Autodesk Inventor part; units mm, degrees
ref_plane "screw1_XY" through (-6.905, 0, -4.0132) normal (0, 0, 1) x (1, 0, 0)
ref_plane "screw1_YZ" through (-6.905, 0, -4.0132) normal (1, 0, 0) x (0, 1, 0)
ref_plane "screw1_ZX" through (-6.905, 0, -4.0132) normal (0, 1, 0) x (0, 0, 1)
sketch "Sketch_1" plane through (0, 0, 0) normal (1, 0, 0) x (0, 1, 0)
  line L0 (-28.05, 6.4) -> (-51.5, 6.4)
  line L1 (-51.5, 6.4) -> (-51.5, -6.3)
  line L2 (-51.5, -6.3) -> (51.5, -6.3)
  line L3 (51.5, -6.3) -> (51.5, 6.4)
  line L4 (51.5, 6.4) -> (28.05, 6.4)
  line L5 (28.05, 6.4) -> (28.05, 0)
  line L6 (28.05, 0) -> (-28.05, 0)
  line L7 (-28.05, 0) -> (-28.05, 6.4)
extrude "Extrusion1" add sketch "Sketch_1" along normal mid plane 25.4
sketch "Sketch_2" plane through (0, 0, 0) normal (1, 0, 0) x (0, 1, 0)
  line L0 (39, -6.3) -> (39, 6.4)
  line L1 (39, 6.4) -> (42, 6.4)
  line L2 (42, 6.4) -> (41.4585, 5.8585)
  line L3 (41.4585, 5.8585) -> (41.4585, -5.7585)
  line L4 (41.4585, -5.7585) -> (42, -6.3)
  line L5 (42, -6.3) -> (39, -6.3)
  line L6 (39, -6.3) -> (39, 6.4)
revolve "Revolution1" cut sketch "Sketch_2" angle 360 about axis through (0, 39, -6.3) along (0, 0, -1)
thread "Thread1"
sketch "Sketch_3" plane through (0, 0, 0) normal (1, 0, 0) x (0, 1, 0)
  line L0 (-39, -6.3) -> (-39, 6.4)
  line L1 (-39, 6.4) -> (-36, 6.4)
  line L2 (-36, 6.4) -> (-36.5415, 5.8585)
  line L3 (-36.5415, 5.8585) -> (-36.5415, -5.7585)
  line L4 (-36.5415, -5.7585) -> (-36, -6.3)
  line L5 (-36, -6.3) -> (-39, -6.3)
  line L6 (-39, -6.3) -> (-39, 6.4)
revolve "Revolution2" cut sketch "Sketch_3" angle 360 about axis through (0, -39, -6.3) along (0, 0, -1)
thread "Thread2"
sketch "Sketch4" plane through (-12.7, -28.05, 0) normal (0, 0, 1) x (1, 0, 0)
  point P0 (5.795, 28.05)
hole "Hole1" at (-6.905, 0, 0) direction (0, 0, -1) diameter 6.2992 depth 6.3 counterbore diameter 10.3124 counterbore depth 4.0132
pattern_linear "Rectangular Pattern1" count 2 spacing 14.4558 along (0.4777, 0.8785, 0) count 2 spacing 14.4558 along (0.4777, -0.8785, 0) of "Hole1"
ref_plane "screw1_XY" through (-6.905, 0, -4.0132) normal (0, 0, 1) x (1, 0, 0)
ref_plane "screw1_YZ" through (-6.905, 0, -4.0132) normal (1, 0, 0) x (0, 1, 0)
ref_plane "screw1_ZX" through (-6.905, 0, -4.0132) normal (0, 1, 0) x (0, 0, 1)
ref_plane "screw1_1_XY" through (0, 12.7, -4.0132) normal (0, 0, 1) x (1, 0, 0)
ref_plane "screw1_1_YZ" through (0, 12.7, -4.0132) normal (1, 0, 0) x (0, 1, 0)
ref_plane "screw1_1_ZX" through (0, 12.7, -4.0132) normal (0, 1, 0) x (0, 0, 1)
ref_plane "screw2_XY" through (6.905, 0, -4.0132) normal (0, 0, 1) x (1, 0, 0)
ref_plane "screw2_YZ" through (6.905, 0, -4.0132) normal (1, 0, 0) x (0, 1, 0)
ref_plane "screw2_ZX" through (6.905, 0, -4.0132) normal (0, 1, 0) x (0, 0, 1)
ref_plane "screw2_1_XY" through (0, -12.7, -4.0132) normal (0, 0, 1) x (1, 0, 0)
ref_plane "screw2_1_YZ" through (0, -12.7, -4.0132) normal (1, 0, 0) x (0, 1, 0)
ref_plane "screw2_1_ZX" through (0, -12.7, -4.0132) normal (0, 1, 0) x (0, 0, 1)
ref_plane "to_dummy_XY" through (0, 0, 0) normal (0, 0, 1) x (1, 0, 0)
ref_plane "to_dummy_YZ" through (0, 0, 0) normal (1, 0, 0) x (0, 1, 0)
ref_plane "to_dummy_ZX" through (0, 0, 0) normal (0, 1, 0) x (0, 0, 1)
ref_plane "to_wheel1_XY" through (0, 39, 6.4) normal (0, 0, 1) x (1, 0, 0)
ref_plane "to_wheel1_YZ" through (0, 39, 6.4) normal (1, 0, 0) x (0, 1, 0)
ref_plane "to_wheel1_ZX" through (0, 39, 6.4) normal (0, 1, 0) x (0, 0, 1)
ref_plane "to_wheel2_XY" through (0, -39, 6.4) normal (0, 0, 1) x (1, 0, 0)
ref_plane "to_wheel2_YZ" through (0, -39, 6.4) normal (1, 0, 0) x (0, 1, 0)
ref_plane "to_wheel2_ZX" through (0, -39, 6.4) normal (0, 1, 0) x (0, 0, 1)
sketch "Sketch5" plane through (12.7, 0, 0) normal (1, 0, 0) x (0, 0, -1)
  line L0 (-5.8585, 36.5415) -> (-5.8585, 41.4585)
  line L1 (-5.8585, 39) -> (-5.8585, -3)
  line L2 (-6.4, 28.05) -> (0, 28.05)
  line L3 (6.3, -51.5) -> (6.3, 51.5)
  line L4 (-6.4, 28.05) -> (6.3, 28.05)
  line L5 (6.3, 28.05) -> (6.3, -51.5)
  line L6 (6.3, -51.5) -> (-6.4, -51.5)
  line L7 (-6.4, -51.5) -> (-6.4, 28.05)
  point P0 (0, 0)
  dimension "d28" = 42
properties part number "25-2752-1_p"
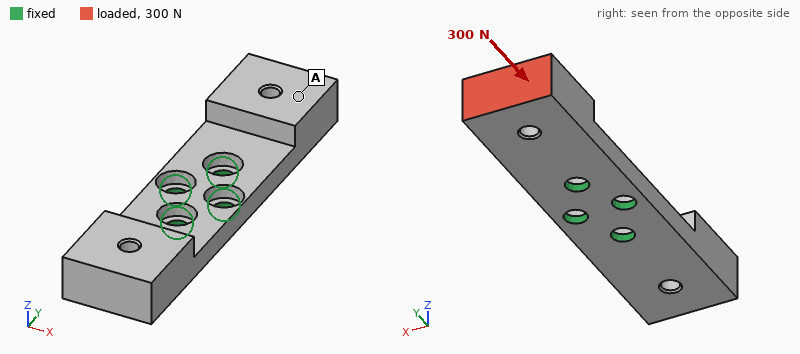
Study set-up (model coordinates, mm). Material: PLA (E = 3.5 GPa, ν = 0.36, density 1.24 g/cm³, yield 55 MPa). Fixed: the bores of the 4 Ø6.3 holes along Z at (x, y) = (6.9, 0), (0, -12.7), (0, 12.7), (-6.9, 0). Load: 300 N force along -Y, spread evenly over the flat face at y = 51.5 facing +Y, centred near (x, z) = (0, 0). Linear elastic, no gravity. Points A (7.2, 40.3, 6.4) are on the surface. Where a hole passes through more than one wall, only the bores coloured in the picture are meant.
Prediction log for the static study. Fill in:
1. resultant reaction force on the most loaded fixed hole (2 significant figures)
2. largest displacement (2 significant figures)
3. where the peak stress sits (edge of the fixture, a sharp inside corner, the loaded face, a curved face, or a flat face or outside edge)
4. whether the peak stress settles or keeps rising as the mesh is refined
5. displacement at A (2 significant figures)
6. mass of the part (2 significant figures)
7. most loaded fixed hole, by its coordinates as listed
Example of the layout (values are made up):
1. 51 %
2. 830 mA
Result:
1. 130 N
2. 0.47 mm
3. edge of the fixture
4. keeps rising
5. 0.33 mm
6. 27 g
7. (0, 12.7)
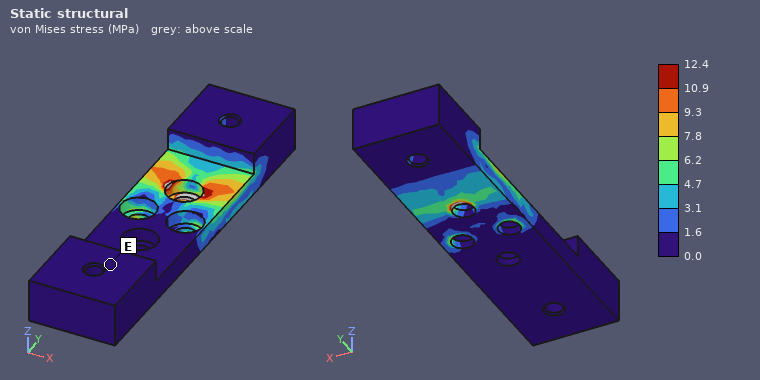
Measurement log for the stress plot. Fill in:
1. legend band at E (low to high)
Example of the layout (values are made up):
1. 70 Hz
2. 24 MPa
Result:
1. 0.0 to 1.6 MPa
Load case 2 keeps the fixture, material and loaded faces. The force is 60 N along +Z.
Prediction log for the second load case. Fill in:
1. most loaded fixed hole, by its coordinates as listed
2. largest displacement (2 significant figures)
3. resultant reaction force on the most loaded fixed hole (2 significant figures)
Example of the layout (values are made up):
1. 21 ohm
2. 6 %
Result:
1. (0, 12.7)
2. 0.80 mm
3. 270 N
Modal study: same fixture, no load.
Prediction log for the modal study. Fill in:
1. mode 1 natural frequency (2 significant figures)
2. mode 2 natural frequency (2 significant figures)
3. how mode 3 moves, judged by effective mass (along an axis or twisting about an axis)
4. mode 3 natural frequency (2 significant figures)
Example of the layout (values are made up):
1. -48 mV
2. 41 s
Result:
1. 670 Hz
2. 670 Hz
3. twisting about Z
4. 1600 Hz
